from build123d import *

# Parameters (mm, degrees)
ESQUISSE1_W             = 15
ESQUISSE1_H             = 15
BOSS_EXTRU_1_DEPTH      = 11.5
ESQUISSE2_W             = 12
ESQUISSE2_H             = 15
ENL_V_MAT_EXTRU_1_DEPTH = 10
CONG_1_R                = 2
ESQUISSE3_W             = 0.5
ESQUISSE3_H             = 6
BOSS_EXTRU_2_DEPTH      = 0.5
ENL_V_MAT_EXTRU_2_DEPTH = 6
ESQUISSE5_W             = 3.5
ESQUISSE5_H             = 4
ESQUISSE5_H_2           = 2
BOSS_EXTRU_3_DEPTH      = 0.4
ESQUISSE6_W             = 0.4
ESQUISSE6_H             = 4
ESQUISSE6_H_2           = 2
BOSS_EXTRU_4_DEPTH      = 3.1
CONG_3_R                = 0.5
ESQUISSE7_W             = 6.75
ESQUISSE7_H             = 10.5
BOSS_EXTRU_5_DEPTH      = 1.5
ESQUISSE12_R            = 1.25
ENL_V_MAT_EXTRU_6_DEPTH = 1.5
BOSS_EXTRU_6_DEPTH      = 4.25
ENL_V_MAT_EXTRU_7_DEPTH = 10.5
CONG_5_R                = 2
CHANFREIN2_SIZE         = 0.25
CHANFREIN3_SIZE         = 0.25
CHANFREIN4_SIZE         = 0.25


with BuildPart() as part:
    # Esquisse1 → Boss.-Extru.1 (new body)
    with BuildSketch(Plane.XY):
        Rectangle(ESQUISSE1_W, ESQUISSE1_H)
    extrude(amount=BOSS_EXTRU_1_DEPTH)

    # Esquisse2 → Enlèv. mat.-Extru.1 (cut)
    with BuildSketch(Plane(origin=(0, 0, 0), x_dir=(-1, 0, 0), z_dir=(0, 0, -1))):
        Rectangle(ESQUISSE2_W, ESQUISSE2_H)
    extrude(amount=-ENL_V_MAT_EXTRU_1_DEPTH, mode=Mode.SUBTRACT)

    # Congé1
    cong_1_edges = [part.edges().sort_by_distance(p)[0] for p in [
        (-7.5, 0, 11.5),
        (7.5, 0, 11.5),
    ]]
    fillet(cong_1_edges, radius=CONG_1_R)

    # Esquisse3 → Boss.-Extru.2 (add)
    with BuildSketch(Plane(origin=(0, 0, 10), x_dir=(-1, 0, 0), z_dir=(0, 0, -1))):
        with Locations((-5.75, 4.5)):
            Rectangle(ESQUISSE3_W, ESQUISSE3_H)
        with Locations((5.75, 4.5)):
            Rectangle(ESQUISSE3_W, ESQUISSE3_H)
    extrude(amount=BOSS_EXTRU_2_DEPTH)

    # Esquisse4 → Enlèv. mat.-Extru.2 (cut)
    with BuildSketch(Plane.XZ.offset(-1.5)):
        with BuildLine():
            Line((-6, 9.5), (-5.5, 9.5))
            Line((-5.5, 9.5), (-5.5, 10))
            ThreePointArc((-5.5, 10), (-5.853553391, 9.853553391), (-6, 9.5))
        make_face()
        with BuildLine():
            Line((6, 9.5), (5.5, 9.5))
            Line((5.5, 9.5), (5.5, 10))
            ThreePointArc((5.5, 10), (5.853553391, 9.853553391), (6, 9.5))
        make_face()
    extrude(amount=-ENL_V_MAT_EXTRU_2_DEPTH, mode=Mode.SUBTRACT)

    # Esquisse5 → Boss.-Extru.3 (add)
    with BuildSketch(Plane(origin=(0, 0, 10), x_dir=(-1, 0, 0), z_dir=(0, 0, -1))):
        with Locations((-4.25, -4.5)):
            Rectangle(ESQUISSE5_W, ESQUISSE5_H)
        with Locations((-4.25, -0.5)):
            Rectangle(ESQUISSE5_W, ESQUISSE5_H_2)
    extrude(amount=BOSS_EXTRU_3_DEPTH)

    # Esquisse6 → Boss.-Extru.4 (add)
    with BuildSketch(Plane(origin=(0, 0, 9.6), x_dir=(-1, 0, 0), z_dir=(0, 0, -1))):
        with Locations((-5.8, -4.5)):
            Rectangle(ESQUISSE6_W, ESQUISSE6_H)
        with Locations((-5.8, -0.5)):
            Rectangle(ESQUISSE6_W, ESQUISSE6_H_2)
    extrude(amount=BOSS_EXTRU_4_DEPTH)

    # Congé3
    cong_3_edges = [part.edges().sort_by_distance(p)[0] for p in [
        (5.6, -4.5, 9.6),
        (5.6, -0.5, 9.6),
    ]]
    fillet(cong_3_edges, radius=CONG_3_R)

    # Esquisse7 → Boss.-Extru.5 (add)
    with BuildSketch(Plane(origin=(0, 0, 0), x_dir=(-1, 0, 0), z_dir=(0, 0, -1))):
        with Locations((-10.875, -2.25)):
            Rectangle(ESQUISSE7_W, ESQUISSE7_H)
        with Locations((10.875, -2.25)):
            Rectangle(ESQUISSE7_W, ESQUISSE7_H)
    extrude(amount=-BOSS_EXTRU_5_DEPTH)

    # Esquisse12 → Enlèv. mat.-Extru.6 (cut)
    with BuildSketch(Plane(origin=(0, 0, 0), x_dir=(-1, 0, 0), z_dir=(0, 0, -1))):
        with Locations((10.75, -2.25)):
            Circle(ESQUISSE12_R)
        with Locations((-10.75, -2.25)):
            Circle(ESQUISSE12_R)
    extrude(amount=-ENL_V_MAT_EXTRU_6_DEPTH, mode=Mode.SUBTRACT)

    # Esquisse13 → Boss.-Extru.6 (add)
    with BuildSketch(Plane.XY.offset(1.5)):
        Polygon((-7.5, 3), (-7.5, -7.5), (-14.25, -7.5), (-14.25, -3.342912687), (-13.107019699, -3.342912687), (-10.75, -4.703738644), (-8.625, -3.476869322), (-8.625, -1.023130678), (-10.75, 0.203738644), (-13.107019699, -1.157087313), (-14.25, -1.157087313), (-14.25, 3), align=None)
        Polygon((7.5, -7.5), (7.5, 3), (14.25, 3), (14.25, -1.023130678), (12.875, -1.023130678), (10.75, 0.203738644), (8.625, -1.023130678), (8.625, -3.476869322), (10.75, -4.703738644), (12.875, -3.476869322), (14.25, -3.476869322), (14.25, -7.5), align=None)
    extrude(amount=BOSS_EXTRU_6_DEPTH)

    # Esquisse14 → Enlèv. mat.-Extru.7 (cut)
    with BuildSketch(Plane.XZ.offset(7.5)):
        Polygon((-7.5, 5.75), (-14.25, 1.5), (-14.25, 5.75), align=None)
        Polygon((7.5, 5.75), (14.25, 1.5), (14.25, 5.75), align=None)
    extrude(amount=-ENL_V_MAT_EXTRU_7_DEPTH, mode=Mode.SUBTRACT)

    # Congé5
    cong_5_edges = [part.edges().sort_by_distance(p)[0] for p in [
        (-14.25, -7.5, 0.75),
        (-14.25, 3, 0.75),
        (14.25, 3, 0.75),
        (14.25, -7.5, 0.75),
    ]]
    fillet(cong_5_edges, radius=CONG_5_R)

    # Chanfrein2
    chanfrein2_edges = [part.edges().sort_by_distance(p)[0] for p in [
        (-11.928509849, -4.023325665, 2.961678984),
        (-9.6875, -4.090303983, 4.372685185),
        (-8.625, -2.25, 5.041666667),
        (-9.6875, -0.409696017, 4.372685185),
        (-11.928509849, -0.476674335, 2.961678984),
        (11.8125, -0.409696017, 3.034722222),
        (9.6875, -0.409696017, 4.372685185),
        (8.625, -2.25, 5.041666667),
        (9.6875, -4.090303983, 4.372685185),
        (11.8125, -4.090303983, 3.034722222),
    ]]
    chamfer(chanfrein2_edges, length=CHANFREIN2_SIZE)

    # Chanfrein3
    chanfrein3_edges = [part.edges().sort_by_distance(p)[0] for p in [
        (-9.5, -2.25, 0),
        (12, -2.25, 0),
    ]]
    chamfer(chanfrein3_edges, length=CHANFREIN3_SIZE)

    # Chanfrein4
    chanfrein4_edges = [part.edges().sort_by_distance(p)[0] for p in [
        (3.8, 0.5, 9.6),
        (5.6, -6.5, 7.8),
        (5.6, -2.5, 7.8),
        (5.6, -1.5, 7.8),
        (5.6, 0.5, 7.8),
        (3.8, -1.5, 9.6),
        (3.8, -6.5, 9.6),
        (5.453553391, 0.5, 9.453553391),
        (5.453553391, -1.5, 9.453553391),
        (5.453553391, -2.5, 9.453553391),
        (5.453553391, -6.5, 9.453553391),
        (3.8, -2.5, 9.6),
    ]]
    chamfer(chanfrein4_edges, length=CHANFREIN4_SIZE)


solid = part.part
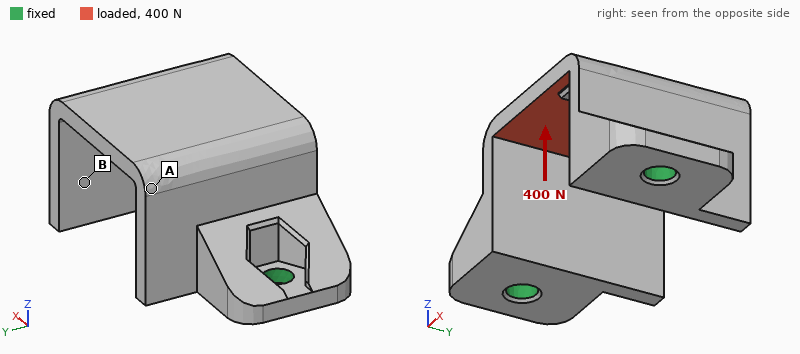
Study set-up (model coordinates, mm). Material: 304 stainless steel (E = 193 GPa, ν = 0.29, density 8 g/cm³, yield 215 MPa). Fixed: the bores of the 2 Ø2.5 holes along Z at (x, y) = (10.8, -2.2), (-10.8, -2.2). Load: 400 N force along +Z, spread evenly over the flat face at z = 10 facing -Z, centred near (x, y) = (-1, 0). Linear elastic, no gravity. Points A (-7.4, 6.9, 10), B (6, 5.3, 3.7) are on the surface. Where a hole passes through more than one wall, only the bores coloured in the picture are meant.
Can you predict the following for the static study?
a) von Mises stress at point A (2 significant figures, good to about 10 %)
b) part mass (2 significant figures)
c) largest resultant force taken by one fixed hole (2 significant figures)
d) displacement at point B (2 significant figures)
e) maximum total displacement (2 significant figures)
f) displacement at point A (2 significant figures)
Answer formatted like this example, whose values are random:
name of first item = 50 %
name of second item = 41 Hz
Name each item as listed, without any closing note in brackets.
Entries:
von Mises stress at point A = 38 MPa
part mass = 9.6 g
largest resultant force taken by one fixed hole = 240 N
displacement at point B = 6.4 µm
maximum total displacement = 17 µm
displacement at point A = 9.6 µm
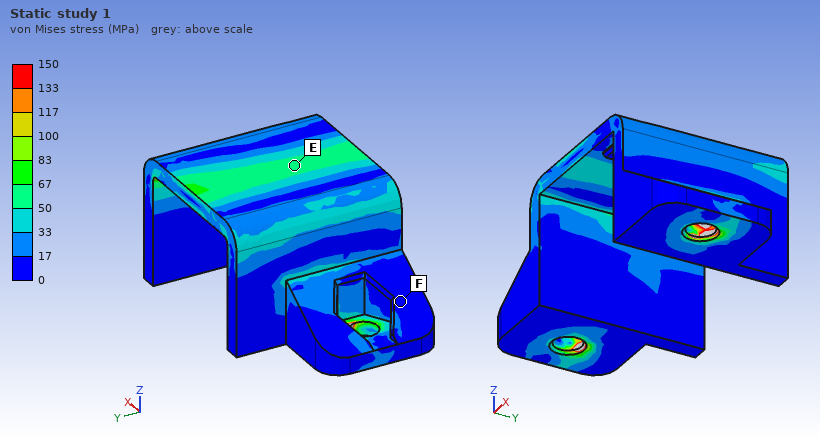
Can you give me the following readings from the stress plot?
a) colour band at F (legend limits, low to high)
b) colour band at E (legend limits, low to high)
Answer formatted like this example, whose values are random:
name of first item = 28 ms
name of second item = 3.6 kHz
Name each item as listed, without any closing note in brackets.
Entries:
colour band at F = 0 to 17 MPa
colour band at E = 50 to 67 MPa
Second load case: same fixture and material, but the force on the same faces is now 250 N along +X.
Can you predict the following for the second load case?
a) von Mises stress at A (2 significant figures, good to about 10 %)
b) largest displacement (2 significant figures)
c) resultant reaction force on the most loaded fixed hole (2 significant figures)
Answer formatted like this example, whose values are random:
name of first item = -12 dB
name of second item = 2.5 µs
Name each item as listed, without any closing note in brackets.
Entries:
von Mises stress at A = 38 MPa
largest displacement = 13 µm
resultant reaction force on the most loaded fixed hole = 140 N
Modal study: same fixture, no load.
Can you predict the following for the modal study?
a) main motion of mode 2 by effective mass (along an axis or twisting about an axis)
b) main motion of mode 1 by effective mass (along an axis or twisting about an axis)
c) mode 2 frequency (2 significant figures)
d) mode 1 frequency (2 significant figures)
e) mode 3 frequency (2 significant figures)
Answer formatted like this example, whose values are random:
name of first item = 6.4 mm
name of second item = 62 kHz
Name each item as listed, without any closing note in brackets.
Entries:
main motion of mode 2 by effective mass = along X
main motion of mode 1 by effective mass = along Y
mode 2 frequency = 12 kHz
mode 1 frequency = 8100 Hz
mode 3 frequency = 15 kHz
